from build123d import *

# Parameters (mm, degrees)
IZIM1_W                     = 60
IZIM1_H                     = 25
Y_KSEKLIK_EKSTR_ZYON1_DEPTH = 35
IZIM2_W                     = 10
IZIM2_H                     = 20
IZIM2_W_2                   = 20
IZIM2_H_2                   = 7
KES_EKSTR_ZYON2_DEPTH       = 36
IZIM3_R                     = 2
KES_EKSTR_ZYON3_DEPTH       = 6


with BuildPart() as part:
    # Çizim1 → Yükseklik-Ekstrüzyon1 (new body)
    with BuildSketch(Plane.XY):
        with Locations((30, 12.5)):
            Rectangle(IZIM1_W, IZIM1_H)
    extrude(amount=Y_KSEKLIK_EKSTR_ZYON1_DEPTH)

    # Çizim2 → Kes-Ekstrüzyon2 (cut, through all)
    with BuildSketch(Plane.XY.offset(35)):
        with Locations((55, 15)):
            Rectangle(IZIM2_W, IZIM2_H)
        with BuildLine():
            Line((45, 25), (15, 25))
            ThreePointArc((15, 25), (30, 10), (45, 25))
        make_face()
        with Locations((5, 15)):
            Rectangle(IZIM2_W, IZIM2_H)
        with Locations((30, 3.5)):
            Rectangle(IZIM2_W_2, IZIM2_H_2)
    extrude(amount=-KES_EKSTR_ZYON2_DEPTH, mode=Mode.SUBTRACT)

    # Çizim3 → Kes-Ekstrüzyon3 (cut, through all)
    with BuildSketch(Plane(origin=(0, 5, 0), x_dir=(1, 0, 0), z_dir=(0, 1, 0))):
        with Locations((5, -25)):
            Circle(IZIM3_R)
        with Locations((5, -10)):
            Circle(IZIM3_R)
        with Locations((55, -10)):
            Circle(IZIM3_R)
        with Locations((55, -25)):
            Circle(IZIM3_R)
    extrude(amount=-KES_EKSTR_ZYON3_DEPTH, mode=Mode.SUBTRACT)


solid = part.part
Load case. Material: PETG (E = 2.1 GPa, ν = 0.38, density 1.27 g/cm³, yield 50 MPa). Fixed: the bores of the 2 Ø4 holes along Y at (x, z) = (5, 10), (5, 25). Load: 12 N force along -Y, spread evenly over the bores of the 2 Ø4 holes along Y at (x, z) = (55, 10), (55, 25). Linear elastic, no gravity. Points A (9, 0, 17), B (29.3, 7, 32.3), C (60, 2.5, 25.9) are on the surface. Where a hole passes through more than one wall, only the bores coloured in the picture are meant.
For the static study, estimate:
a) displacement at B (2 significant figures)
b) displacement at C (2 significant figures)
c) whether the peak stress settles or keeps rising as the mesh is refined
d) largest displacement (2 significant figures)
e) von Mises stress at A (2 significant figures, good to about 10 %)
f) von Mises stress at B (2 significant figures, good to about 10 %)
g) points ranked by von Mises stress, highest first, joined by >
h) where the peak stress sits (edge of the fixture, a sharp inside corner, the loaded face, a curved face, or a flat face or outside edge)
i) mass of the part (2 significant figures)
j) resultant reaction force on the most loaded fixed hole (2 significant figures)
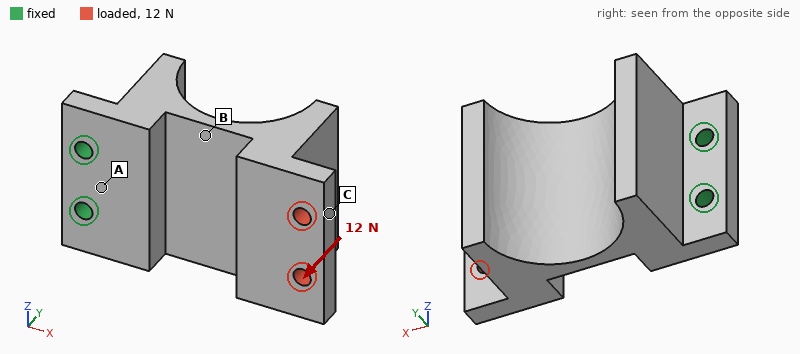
0.15 mm
0.87 mm
keeps rising
0.89 mm
2.8 MPa
5.1 MPa
B > A > C
edge of the fixture
27 g
6.0 N
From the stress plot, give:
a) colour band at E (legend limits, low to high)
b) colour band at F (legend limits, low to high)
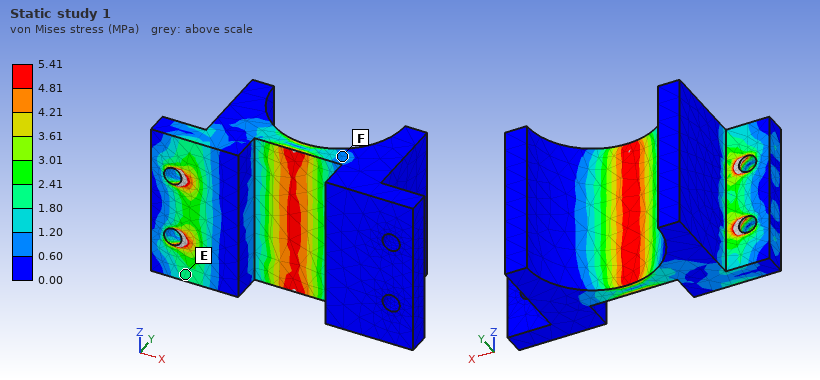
1.80 to 2.41 MPa
0.60 to 1.20 MPa
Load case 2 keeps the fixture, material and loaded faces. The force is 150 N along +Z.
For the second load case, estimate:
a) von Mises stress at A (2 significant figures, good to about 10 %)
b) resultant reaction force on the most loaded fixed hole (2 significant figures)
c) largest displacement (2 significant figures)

6.5 MPa
420 N
0.78 mm
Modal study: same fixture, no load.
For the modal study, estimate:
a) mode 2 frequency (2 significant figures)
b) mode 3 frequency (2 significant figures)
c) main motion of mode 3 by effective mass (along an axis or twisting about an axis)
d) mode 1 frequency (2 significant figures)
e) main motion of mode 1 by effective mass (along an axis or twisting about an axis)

870 Hz
980 Hz
along Z
230 Hz
along Y
